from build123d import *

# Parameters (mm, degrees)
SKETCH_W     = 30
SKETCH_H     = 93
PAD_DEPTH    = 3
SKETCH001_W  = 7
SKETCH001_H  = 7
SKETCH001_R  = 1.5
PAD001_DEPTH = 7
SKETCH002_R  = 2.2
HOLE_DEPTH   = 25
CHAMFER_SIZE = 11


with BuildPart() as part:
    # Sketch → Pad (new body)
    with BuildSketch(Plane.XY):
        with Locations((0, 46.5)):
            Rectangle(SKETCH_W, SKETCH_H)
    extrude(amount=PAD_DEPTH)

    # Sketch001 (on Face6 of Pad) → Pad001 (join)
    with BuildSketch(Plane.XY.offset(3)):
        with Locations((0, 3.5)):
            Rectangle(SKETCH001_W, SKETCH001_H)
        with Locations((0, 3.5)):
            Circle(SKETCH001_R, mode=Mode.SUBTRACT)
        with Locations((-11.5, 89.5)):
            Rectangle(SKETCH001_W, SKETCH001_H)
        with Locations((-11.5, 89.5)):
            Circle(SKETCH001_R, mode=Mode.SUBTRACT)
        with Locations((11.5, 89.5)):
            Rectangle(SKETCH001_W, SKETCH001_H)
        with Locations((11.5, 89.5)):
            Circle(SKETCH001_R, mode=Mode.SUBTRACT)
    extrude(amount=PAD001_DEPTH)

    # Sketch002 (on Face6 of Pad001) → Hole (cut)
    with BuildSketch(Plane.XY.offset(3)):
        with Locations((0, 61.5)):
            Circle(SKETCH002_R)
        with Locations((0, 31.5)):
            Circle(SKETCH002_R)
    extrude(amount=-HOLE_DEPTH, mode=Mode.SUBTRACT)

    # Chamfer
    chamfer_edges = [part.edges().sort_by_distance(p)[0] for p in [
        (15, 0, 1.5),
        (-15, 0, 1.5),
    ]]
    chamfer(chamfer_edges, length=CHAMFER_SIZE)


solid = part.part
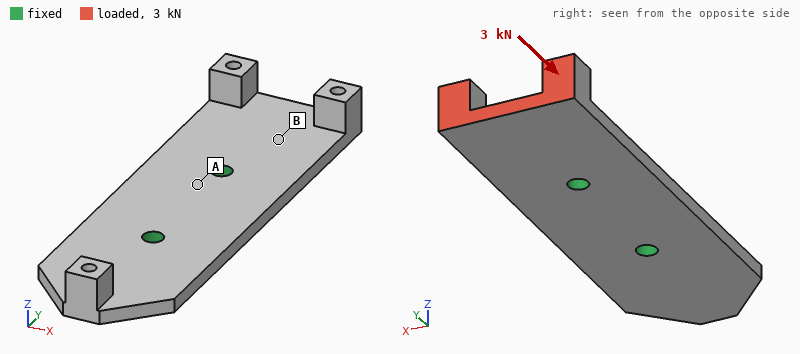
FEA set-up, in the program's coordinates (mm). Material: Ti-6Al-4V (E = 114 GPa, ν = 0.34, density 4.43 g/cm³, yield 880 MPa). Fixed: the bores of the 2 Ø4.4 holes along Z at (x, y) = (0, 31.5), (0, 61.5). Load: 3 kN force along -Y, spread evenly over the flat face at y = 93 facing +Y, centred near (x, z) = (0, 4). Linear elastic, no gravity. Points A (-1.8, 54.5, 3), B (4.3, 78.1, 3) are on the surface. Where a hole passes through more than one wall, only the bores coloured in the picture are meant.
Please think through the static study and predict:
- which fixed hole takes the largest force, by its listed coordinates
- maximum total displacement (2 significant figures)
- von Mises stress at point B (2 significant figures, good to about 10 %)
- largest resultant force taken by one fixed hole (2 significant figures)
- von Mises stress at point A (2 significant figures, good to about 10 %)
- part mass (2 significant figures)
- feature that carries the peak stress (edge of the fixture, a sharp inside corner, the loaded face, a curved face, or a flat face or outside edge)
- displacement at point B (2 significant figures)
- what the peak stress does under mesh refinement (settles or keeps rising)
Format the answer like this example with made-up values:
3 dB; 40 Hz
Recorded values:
(0, 61.5); 0.54 mm; 190 MPa; 2.4 kN; 31 MPa; 39 g; edge of the fixture; 0.15 mm; keeps rising
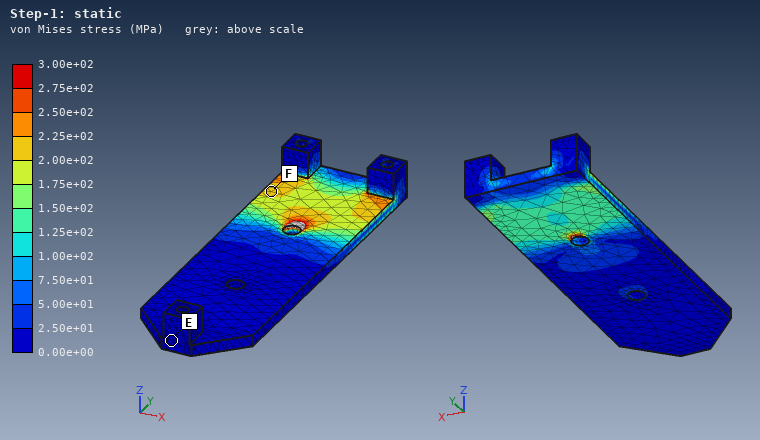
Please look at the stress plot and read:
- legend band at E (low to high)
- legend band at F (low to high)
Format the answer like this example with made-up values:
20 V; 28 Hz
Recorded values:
0.00e+00 to 2.50e+01 MPa; 2.00e+02 to 2.25e+02 MPa
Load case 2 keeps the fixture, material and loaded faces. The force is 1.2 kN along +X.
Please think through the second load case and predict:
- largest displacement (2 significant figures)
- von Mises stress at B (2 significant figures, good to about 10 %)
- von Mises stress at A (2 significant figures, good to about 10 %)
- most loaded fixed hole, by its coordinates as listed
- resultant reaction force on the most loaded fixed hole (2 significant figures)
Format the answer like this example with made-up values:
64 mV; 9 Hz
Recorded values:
0.16 mm; 83 MPa; 16 MPa; (0, 61.5); 2.2 kN
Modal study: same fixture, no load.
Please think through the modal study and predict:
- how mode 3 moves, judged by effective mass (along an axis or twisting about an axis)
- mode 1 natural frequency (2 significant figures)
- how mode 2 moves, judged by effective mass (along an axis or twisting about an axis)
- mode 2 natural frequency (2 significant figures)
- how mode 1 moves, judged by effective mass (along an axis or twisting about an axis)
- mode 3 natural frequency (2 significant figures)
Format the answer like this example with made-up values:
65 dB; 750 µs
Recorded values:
twisting about Y; 1900 Hz; along Z; 2500 Hz; along Z; 3500 Hz
